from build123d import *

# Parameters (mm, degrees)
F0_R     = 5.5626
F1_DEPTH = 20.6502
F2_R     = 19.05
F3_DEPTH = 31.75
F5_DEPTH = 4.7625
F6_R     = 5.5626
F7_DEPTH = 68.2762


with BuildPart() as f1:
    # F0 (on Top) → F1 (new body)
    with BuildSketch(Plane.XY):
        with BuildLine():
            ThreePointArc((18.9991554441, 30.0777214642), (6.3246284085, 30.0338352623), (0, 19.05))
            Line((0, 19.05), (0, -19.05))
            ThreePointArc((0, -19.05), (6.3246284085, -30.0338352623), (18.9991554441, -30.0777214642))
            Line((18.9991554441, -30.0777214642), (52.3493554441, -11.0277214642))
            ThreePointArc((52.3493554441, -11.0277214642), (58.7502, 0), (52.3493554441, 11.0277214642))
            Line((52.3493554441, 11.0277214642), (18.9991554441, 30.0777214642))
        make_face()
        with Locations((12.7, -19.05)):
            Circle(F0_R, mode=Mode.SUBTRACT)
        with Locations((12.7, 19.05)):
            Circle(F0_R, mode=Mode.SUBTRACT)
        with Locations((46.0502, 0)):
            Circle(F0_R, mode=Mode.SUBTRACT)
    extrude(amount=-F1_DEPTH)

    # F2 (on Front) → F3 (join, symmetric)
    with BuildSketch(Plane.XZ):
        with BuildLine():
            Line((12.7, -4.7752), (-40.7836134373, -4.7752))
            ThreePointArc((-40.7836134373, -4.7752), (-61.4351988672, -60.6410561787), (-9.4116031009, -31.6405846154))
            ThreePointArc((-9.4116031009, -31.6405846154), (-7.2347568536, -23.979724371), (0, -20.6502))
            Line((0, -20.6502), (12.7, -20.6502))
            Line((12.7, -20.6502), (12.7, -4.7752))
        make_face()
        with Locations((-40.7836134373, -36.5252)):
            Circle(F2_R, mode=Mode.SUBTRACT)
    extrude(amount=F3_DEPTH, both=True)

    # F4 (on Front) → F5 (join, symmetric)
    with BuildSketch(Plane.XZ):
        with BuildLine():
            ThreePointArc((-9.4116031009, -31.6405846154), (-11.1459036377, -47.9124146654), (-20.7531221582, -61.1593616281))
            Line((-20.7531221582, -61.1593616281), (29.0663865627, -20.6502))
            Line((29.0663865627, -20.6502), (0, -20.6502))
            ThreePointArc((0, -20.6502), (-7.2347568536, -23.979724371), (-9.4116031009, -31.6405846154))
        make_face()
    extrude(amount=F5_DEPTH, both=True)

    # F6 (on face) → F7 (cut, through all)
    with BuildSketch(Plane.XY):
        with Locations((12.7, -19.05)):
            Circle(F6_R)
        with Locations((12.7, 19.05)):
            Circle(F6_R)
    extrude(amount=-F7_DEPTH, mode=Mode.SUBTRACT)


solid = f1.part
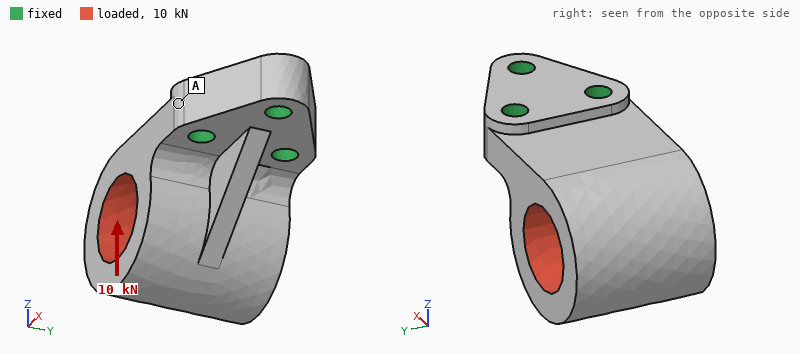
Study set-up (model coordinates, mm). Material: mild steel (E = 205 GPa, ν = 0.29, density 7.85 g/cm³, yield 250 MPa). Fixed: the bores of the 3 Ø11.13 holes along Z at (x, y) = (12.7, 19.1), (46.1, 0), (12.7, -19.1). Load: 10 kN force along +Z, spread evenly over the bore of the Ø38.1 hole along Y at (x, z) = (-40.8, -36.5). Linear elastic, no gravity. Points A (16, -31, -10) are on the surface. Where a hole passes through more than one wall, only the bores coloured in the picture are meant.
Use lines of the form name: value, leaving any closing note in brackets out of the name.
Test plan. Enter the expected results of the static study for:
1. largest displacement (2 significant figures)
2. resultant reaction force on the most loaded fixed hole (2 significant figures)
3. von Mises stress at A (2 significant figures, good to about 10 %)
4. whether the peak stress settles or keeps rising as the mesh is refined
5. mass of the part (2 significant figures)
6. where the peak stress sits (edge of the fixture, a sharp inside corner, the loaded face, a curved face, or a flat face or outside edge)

largest displacement: 96 µm
resultant reaction force on the most loaded fixed hole: 7.0 kN
von Mises stress at A: 16 MPa
whether the peak stress settles or keeps rising as the mesh is refined: keeps rising
mass of the part: 1.6 kg
where the peak stress sits: edge of the fixture
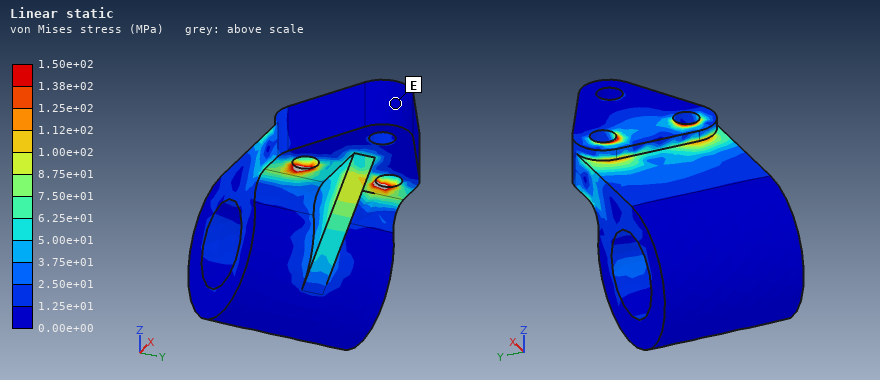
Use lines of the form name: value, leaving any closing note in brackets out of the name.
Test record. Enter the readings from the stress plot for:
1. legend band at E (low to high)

legend band at E: 0.00e+00 to 1.25e+01 MPa
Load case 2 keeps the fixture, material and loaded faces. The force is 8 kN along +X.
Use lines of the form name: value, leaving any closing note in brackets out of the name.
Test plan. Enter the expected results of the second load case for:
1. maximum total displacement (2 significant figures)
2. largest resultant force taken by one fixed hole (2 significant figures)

maximum total displacement: 41 µm
largest resultant force taken by one fixed hole: 3.3 kN
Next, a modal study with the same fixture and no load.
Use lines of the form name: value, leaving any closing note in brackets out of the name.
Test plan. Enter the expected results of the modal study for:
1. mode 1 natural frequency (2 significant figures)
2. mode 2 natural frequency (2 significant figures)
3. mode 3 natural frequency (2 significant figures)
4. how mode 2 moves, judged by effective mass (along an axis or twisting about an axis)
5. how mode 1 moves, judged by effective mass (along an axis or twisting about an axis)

mode 1 natural frequency: 1700 Hz
mode 2 natural frequency: 3200 Hz
mode 3 natural frequency: 5200 Hz
how mode 2 moves, judged by effective mass: along Y
how mode 1 moves, judged by effective mass: along Z
